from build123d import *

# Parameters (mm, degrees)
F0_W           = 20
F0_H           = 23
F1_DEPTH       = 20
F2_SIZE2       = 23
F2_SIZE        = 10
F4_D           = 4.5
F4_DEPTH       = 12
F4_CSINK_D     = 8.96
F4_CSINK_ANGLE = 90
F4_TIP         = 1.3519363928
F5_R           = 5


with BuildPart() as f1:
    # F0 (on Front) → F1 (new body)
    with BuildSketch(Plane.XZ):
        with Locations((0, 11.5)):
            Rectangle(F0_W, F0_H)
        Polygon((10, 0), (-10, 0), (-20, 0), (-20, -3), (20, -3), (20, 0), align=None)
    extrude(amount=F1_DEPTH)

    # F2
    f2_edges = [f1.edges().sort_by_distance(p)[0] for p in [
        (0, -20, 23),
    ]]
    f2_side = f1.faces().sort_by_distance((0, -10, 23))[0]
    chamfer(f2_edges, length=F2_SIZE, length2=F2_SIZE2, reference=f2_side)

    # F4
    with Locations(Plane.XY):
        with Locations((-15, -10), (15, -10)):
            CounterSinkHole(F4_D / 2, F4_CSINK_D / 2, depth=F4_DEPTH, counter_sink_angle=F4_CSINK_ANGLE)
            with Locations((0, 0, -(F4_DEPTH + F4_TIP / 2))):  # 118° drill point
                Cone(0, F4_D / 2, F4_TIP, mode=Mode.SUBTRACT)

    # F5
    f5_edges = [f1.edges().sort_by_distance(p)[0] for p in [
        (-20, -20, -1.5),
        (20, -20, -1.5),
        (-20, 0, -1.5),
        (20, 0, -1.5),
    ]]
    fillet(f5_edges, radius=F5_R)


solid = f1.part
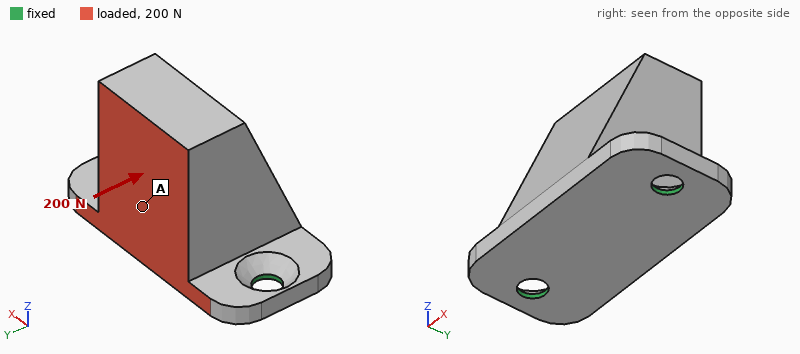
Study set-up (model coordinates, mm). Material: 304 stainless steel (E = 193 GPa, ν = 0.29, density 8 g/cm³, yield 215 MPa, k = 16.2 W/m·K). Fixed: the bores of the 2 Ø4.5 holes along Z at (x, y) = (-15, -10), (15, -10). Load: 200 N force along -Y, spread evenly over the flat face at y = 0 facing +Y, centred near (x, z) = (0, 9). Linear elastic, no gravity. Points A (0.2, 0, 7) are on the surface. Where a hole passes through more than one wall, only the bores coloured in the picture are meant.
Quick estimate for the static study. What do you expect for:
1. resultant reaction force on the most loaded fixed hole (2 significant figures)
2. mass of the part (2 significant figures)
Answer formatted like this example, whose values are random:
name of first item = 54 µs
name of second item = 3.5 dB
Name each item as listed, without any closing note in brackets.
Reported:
resultant reaction force on the most loaded fixed hole = 100 N
mass of the part = 72 g
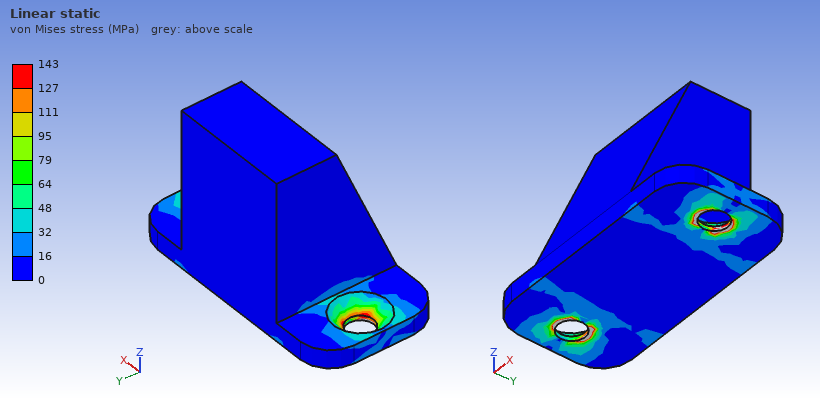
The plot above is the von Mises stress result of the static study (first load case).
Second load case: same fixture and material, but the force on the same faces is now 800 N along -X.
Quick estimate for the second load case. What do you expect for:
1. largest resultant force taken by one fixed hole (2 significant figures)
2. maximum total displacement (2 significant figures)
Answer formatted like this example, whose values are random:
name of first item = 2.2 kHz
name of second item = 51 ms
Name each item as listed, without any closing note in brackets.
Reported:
largest resultant force taken by one fixed hole = 590 N
maximum total displacement = 6.7 µm
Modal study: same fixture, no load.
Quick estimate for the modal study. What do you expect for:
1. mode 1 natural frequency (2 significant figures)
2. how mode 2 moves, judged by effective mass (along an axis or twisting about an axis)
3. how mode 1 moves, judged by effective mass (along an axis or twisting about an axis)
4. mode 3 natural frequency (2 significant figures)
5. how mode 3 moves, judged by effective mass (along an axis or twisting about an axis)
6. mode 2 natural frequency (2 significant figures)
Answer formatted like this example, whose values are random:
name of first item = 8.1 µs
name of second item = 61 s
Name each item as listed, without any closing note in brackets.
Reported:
mode 1 natural frequency = 2000 Hz
how mode 2 moves, judged by effective mass = along X
how mode 1 moves, judged by effective mass = along Y
mode 3 natural frequency = 10 kHz
how mode 3 moves, judged by effective mass = along Z
mode 2 natural frequency = 8900 Hz
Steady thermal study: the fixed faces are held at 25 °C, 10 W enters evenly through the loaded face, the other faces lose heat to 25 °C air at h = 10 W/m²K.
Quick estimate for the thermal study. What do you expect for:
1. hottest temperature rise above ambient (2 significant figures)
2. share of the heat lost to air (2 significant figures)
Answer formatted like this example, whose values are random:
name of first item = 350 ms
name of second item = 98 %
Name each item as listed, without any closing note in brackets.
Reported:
hottest temperature rise above ambient = 75 K
share of the heat lost to air = 13 %
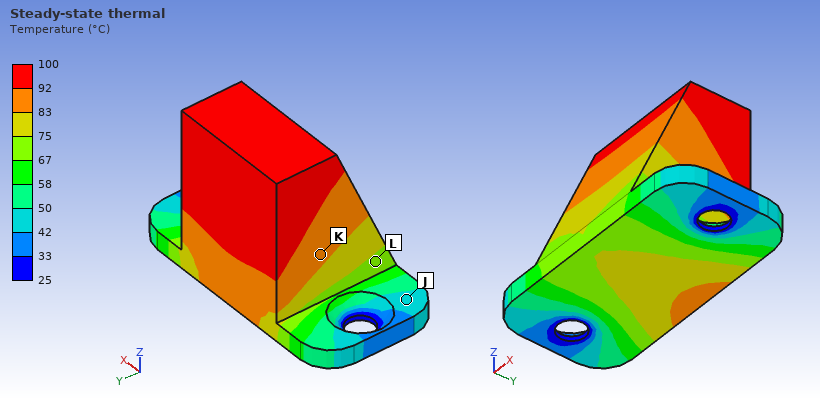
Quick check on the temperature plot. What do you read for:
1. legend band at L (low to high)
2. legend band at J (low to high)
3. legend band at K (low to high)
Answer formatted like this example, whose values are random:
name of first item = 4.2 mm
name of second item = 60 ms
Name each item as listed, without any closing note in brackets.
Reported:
legend band at L = 67 to 75 °C
legend band at J = 42 to 50 °C
legend band at K = 83 to 92 °C
